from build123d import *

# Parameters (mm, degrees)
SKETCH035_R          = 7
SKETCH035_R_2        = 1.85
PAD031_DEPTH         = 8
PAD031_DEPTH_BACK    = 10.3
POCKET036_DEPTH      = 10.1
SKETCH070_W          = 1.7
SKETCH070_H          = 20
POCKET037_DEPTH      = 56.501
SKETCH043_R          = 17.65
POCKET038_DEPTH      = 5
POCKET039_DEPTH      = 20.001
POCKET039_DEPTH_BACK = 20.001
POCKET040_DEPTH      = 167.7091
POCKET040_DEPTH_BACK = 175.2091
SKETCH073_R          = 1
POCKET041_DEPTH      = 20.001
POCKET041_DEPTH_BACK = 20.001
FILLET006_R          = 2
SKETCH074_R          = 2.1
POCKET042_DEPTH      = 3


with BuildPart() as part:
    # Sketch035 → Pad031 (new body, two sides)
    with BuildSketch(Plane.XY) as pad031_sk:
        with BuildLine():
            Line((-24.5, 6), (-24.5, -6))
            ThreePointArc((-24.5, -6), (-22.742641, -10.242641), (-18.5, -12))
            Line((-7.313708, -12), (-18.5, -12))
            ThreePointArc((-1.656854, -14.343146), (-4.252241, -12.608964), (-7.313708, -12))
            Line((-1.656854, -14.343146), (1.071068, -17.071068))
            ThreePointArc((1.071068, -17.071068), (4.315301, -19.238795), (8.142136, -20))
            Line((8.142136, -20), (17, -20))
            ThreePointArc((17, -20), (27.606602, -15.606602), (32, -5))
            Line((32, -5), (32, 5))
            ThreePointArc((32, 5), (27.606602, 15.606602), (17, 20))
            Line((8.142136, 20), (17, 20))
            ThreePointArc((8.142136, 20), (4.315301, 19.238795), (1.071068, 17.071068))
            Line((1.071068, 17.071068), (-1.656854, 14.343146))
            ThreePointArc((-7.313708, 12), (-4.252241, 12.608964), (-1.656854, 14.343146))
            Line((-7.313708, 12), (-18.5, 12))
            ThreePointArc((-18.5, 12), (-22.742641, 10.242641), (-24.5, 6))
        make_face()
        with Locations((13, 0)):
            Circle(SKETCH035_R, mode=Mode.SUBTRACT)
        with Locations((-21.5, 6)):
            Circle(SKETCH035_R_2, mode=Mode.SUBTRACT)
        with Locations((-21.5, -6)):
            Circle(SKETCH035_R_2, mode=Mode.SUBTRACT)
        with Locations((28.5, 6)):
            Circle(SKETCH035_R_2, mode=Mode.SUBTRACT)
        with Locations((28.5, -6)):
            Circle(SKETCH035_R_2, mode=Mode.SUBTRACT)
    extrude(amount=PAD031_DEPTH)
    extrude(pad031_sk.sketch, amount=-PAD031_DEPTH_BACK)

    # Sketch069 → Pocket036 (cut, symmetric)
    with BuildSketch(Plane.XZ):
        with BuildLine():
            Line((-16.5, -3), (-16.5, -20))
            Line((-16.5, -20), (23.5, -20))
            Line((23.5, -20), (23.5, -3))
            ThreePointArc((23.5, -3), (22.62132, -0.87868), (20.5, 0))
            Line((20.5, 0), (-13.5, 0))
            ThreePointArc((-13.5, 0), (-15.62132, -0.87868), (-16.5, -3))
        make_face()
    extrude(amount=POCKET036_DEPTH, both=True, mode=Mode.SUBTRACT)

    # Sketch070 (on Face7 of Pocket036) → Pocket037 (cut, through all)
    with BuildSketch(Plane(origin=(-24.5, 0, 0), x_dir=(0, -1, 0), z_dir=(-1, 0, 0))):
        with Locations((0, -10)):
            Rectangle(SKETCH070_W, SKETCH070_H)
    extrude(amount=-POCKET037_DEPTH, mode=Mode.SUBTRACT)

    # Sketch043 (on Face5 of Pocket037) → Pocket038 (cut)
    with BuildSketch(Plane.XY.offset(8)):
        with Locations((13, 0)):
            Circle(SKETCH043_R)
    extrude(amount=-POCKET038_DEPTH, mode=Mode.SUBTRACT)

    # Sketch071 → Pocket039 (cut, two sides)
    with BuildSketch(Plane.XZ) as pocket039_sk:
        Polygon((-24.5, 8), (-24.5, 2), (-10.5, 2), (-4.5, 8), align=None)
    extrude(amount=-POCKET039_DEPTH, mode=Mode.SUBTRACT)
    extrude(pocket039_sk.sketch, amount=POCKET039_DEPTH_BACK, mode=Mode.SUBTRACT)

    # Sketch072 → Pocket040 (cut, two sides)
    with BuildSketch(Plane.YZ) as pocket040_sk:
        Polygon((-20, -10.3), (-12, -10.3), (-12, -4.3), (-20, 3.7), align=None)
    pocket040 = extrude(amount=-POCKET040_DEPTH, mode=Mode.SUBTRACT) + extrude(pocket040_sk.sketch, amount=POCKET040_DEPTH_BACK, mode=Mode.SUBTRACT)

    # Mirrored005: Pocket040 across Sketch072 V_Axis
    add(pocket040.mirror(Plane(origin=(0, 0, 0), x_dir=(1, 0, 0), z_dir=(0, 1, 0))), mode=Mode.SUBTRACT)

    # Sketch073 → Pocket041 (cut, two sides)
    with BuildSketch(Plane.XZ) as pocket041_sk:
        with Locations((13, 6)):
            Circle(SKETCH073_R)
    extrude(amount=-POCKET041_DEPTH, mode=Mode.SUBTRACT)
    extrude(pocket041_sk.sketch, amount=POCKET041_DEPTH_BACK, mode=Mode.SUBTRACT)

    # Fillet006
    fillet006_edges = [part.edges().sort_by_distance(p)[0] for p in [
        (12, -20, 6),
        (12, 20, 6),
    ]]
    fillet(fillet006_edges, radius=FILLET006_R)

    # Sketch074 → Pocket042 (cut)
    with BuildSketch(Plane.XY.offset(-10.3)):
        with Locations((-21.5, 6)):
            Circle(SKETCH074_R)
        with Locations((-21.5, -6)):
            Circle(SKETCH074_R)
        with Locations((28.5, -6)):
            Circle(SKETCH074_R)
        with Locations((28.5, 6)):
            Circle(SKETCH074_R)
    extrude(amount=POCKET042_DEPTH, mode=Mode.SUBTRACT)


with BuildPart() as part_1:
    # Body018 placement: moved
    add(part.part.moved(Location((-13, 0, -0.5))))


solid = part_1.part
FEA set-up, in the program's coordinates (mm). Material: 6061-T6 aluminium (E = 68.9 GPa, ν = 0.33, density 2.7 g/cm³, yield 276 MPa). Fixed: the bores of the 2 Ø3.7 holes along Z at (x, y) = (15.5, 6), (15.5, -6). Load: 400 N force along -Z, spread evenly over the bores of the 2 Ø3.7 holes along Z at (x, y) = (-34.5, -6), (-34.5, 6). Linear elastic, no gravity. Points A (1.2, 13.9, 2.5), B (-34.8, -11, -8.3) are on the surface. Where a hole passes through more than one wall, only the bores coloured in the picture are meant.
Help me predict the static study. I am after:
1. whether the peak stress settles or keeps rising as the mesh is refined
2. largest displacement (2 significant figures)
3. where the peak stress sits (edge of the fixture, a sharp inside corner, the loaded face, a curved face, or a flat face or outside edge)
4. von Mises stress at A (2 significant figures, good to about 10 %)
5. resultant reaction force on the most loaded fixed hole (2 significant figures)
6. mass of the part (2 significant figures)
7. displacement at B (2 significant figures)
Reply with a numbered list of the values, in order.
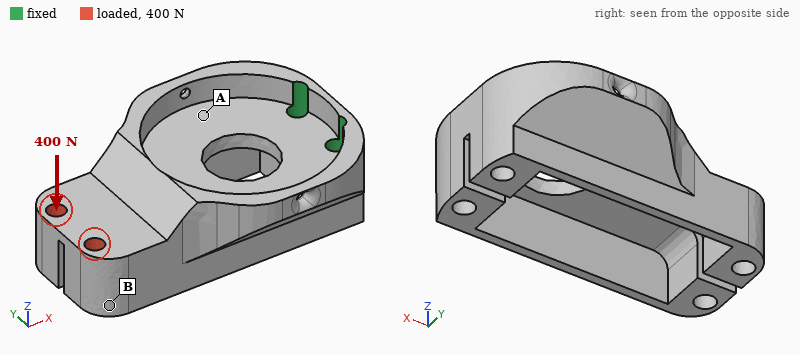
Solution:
1. keeps rising
2. 0.20 mm
3. edge of the fixture
4. 25 MPa
5. 200 N
6. 30 g
7. 0.17 mm
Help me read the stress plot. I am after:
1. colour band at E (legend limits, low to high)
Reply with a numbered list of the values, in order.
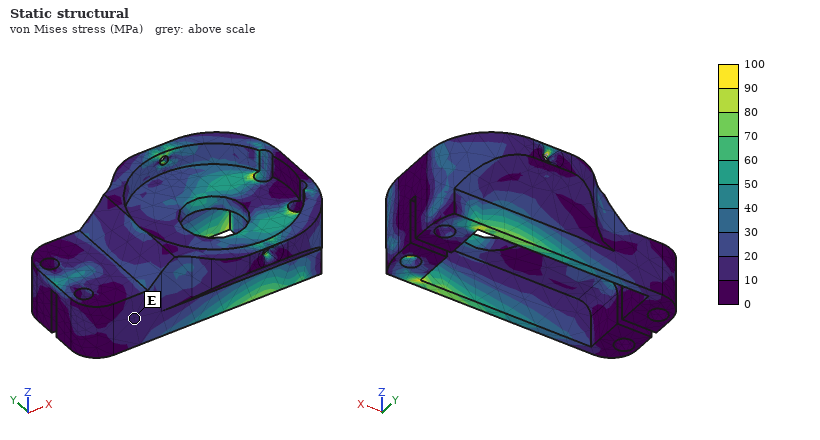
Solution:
1. 10 to 20 MPa
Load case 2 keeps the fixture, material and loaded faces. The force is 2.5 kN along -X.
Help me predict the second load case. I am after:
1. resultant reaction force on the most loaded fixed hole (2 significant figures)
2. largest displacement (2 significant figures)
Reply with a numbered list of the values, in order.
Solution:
1. 1.3 kN
2. 76 µm
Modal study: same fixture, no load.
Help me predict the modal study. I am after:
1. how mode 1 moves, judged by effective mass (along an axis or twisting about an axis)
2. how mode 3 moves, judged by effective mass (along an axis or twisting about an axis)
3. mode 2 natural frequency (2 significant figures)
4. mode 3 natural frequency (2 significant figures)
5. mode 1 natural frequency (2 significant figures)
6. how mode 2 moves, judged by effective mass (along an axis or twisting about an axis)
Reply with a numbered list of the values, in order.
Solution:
1. along Z
2. along Y
3. 4200 Hz
4. 6600 Hz
5. 2800 Hz
6. along Y
